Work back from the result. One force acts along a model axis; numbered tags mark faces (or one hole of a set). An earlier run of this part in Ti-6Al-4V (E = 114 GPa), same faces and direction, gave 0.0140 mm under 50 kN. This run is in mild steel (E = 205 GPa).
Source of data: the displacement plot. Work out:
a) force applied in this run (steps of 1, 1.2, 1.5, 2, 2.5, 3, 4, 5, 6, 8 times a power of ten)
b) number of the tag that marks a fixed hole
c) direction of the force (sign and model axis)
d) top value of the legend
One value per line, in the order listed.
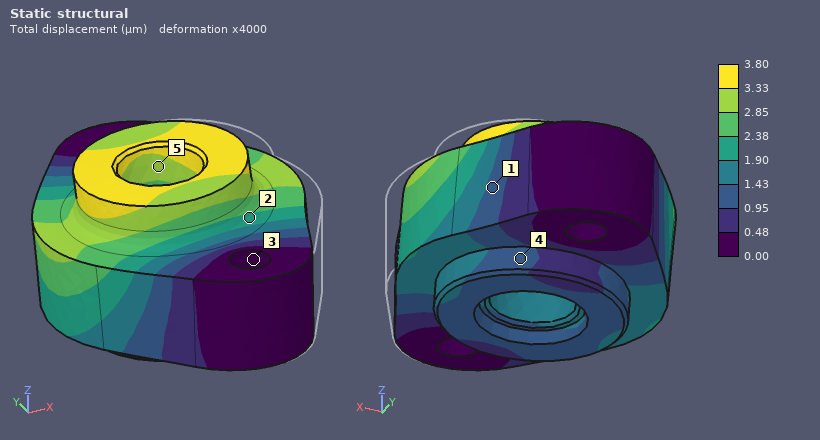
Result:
25 kN
3
-X
3.80 µm
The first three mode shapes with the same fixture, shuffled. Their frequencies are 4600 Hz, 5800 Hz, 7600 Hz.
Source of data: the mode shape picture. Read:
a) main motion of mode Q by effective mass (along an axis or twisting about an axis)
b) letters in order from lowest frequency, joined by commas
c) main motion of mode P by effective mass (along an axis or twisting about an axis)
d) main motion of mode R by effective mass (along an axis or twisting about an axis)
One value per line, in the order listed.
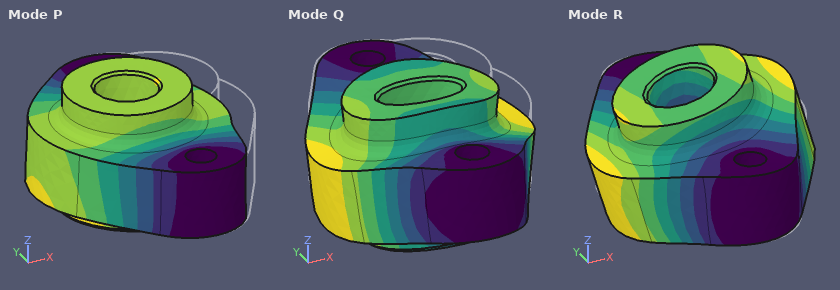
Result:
along Z
R, Q, P
along X
twisting about Y
